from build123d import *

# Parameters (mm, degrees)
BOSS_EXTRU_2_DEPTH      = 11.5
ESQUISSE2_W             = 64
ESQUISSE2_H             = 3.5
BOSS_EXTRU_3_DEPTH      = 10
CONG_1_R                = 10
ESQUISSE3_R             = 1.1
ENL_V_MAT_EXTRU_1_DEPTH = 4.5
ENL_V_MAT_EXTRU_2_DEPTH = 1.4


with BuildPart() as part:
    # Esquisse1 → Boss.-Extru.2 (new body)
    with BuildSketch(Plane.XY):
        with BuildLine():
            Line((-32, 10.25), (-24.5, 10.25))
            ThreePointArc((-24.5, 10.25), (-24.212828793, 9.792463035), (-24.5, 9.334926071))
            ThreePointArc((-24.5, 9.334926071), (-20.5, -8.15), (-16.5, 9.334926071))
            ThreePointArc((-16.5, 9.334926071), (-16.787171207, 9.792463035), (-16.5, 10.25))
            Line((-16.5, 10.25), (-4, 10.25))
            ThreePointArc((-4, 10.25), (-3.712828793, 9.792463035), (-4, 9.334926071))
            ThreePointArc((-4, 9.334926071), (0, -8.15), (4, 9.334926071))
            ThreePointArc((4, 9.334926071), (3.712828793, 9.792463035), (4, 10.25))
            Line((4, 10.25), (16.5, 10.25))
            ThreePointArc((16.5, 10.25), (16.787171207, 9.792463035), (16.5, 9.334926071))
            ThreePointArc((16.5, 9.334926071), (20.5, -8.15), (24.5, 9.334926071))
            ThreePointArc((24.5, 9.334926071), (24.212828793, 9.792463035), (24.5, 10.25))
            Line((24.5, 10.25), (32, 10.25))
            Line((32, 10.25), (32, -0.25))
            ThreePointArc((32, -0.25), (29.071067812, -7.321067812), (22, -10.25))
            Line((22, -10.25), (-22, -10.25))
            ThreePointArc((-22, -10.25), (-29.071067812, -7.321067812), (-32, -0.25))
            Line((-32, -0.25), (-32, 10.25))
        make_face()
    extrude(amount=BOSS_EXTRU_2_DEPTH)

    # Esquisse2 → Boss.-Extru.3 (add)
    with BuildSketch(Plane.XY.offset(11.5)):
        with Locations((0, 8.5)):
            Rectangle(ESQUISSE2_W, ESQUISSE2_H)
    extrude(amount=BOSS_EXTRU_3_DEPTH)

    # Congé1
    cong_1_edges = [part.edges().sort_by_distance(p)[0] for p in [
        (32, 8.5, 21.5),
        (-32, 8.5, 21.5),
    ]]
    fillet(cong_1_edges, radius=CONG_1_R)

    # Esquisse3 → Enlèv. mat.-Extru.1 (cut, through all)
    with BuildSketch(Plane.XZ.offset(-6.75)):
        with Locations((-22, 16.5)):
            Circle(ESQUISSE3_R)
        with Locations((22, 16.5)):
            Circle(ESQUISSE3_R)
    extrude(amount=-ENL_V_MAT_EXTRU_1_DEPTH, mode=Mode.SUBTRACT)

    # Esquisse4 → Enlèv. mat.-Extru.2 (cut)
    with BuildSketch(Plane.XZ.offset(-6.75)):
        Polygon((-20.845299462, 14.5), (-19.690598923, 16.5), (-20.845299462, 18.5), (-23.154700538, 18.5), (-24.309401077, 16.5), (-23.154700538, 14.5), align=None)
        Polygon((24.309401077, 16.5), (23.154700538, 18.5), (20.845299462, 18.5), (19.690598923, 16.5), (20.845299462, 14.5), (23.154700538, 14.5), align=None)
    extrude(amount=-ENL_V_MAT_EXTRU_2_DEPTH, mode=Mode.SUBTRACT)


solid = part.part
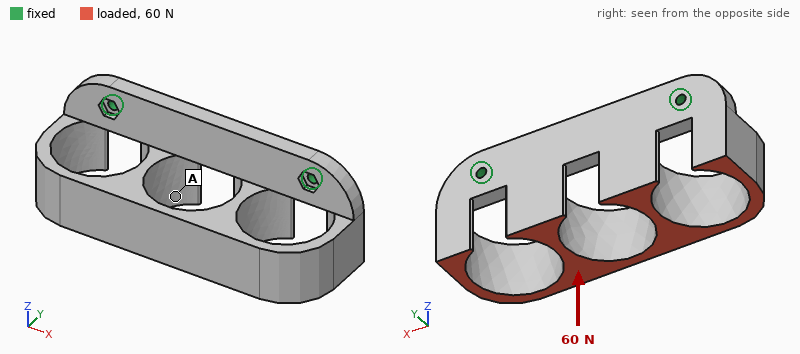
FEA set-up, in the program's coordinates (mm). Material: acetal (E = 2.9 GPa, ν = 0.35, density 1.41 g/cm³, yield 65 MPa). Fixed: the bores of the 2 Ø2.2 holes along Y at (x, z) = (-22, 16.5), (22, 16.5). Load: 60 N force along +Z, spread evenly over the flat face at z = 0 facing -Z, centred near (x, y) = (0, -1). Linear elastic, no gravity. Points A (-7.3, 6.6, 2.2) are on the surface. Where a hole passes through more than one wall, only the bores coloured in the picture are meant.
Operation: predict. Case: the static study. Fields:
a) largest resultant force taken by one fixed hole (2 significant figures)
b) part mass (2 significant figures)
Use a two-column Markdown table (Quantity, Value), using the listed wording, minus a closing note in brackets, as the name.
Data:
| Quantity | Value |
|---|---|
| largest resultant force taken by one fixed hole | 30 N |
| part mass | 10 g |
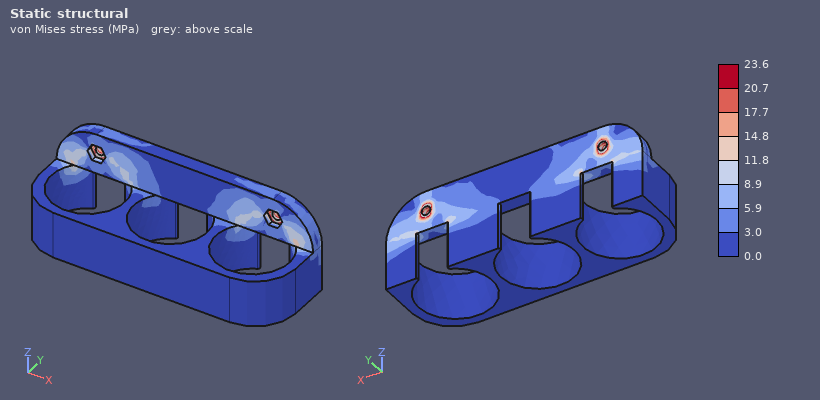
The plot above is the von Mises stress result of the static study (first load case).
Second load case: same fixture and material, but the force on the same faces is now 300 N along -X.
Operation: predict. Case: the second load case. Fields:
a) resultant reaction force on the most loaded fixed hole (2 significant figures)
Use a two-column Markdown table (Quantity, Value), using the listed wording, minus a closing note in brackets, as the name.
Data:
| Quantity | Value |
|---|---|
| resultant reaction force on the most loaded fixed hole | 200 N |
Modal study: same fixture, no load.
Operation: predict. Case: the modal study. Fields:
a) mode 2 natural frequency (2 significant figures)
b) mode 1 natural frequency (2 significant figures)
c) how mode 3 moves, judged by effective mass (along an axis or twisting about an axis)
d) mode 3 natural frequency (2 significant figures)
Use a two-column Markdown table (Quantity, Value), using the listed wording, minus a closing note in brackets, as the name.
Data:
| Quantity | Value |
|---|---|
| mode 2 natural frequency | 1100 Hz |
| mode 1 natural frequency | 530 Hz |
| how mode 3 moves, judged by effective mass | along X |
| mode 3 natural frequency | 1700 Hz |
